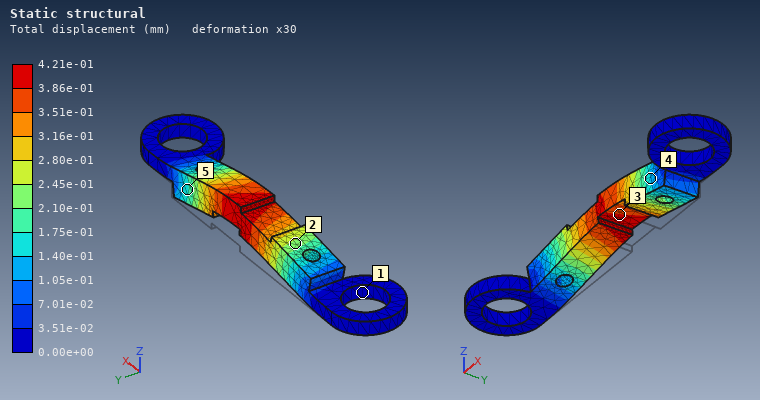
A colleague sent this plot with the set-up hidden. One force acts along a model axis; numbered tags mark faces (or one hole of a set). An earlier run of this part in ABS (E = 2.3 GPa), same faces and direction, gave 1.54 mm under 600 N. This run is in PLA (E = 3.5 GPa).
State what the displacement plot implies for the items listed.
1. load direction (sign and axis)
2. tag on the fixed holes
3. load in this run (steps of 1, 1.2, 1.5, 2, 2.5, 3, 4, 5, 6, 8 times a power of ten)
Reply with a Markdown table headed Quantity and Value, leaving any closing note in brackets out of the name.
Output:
| Quantity | Value |
|---|---|
| load direction | +Z |
| tag on the fixed holes | 1 |
| load in this run | 250 N |
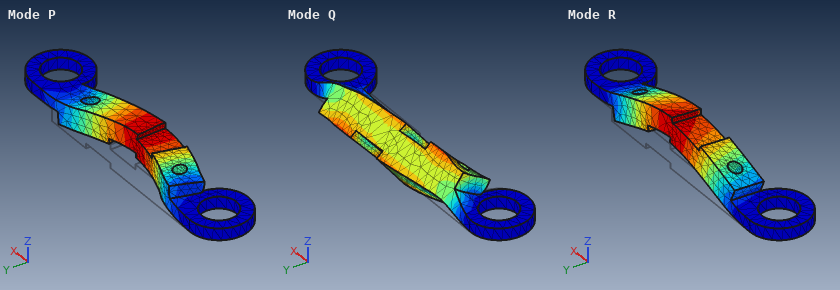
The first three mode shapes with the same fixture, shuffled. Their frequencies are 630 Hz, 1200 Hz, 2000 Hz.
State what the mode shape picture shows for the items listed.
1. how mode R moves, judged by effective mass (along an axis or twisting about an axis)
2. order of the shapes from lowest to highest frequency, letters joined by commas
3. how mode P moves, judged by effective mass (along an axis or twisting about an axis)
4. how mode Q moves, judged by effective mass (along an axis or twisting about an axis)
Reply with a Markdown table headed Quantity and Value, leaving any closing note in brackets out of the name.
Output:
| Quantity | Value |
|---|---|
| how mode R moves, judged by effective mass | along Z |
| order of the shapes from lowest to highest frequency, letters joined by commas | R, P, Q |
| how mode P moves, judged by effective mass | along Y |
| how mode Q moves, judged by effective mass | twisting about X |
